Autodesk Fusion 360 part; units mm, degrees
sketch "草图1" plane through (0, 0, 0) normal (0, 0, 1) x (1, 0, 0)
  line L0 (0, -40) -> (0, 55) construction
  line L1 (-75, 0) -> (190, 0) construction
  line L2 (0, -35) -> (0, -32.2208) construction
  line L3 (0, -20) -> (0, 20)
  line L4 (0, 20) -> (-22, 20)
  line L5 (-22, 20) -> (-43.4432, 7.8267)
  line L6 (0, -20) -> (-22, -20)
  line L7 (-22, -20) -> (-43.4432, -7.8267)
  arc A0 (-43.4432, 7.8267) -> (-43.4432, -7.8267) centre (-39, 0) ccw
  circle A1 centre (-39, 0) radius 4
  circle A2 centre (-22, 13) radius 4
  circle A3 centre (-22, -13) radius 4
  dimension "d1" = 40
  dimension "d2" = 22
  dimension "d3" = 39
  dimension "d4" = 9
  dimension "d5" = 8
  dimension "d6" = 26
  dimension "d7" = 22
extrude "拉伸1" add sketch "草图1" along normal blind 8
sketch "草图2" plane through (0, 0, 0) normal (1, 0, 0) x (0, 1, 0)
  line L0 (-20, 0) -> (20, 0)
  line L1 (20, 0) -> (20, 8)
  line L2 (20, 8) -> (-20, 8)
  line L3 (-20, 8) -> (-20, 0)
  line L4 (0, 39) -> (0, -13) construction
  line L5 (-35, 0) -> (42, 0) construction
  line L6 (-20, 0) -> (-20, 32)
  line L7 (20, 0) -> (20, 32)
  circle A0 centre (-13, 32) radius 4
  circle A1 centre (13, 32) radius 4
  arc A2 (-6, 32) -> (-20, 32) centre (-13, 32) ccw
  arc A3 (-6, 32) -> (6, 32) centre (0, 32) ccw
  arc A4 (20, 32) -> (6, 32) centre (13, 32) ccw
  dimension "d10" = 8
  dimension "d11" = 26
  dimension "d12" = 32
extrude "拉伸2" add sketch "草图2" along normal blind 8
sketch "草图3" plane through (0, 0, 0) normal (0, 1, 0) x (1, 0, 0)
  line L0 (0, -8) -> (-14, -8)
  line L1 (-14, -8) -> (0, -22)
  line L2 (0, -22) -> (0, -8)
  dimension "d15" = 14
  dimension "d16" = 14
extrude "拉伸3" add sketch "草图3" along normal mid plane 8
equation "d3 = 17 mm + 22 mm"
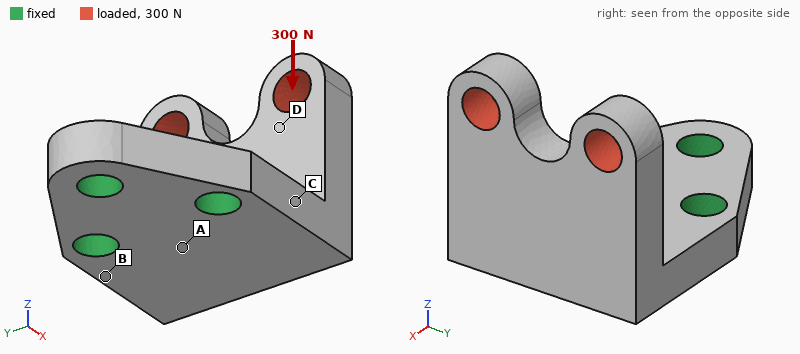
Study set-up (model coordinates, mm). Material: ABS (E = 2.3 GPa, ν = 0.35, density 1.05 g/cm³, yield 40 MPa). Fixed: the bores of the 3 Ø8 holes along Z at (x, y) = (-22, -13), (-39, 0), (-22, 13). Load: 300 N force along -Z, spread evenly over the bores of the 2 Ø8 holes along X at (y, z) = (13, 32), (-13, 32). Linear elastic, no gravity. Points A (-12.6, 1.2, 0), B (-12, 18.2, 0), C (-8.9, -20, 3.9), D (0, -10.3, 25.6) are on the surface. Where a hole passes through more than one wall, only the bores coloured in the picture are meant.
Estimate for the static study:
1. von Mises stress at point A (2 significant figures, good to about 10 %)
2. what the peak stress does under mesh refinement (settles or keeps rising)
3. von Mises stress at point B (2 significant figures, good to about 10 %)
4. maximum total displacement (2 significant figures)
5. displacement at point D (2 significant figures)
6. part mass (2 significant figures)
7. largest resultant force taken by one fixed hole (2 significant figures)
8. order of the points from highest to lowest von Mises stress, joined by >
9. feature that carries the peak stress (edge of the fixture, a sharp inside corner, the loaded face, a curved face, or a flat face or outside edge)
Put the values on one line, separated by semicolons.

8.4 MPa; keeps rising; 11 MPa; 0.77 mm; 0.48 mm; 23 g; 180 N; B > A > C > D; edge of the fixture
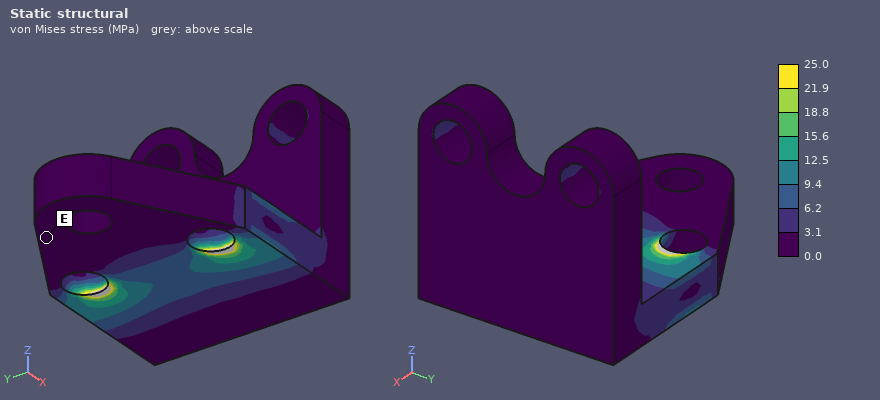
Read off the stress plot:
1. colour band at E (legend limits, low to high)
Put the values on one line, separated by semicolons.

0.0 to 3.1 MPa
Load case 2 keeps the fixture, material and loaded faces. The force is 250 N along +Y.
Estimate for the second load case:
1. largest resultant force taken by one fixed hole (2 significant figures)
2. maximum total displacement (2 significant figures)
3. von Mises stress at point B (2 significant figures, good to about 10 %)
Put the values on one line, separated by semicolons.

350 N; 0.57 mm; 7.0 MPa
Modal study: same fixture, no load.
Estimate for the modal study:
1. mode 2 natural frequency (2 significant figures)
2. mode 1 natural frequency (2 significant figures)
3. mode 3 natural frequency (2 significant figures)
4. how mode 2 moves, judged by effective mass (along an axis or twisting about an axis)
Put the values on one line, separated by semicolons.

1700 Hz; 1000 Hz; 3000 Hz; along Y
